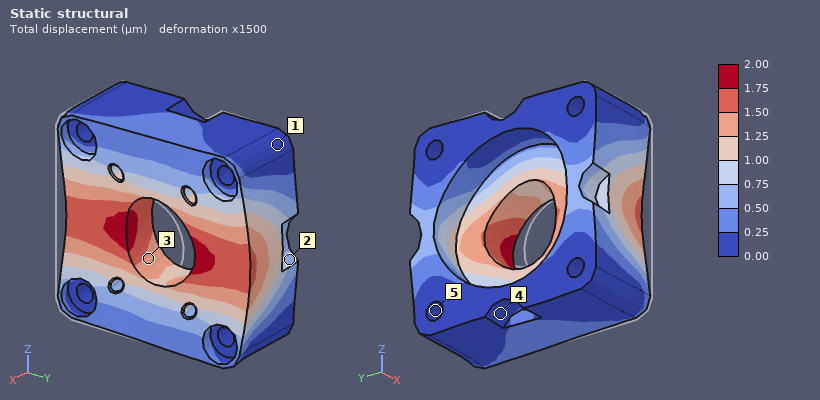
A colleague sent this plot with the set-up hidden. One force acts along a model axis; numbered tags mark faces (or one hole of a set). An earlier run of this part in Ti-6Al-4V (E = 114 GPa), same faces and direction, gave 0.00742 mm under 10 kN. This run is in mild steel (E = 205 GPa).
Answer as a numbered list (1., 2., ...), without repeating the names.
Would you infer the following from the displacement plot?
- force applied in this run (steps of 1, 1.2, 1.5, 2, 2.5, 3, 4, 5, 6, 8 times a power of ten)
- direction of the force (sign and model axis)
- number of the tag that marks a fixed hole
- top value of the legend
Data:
1. 5 kN
2. +Y
3. 5
4. 2.00 µm
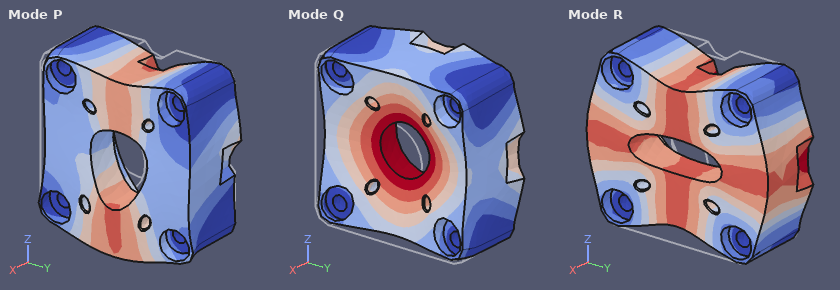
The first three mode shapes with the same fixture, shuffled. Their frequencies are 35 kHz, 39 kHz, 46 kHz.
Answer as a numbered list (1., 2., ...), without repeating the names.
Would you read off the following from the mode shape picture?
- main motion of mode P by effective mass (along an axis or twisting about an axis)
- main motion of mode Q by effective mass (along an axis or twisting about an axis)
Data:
1. along Z
2. along X
